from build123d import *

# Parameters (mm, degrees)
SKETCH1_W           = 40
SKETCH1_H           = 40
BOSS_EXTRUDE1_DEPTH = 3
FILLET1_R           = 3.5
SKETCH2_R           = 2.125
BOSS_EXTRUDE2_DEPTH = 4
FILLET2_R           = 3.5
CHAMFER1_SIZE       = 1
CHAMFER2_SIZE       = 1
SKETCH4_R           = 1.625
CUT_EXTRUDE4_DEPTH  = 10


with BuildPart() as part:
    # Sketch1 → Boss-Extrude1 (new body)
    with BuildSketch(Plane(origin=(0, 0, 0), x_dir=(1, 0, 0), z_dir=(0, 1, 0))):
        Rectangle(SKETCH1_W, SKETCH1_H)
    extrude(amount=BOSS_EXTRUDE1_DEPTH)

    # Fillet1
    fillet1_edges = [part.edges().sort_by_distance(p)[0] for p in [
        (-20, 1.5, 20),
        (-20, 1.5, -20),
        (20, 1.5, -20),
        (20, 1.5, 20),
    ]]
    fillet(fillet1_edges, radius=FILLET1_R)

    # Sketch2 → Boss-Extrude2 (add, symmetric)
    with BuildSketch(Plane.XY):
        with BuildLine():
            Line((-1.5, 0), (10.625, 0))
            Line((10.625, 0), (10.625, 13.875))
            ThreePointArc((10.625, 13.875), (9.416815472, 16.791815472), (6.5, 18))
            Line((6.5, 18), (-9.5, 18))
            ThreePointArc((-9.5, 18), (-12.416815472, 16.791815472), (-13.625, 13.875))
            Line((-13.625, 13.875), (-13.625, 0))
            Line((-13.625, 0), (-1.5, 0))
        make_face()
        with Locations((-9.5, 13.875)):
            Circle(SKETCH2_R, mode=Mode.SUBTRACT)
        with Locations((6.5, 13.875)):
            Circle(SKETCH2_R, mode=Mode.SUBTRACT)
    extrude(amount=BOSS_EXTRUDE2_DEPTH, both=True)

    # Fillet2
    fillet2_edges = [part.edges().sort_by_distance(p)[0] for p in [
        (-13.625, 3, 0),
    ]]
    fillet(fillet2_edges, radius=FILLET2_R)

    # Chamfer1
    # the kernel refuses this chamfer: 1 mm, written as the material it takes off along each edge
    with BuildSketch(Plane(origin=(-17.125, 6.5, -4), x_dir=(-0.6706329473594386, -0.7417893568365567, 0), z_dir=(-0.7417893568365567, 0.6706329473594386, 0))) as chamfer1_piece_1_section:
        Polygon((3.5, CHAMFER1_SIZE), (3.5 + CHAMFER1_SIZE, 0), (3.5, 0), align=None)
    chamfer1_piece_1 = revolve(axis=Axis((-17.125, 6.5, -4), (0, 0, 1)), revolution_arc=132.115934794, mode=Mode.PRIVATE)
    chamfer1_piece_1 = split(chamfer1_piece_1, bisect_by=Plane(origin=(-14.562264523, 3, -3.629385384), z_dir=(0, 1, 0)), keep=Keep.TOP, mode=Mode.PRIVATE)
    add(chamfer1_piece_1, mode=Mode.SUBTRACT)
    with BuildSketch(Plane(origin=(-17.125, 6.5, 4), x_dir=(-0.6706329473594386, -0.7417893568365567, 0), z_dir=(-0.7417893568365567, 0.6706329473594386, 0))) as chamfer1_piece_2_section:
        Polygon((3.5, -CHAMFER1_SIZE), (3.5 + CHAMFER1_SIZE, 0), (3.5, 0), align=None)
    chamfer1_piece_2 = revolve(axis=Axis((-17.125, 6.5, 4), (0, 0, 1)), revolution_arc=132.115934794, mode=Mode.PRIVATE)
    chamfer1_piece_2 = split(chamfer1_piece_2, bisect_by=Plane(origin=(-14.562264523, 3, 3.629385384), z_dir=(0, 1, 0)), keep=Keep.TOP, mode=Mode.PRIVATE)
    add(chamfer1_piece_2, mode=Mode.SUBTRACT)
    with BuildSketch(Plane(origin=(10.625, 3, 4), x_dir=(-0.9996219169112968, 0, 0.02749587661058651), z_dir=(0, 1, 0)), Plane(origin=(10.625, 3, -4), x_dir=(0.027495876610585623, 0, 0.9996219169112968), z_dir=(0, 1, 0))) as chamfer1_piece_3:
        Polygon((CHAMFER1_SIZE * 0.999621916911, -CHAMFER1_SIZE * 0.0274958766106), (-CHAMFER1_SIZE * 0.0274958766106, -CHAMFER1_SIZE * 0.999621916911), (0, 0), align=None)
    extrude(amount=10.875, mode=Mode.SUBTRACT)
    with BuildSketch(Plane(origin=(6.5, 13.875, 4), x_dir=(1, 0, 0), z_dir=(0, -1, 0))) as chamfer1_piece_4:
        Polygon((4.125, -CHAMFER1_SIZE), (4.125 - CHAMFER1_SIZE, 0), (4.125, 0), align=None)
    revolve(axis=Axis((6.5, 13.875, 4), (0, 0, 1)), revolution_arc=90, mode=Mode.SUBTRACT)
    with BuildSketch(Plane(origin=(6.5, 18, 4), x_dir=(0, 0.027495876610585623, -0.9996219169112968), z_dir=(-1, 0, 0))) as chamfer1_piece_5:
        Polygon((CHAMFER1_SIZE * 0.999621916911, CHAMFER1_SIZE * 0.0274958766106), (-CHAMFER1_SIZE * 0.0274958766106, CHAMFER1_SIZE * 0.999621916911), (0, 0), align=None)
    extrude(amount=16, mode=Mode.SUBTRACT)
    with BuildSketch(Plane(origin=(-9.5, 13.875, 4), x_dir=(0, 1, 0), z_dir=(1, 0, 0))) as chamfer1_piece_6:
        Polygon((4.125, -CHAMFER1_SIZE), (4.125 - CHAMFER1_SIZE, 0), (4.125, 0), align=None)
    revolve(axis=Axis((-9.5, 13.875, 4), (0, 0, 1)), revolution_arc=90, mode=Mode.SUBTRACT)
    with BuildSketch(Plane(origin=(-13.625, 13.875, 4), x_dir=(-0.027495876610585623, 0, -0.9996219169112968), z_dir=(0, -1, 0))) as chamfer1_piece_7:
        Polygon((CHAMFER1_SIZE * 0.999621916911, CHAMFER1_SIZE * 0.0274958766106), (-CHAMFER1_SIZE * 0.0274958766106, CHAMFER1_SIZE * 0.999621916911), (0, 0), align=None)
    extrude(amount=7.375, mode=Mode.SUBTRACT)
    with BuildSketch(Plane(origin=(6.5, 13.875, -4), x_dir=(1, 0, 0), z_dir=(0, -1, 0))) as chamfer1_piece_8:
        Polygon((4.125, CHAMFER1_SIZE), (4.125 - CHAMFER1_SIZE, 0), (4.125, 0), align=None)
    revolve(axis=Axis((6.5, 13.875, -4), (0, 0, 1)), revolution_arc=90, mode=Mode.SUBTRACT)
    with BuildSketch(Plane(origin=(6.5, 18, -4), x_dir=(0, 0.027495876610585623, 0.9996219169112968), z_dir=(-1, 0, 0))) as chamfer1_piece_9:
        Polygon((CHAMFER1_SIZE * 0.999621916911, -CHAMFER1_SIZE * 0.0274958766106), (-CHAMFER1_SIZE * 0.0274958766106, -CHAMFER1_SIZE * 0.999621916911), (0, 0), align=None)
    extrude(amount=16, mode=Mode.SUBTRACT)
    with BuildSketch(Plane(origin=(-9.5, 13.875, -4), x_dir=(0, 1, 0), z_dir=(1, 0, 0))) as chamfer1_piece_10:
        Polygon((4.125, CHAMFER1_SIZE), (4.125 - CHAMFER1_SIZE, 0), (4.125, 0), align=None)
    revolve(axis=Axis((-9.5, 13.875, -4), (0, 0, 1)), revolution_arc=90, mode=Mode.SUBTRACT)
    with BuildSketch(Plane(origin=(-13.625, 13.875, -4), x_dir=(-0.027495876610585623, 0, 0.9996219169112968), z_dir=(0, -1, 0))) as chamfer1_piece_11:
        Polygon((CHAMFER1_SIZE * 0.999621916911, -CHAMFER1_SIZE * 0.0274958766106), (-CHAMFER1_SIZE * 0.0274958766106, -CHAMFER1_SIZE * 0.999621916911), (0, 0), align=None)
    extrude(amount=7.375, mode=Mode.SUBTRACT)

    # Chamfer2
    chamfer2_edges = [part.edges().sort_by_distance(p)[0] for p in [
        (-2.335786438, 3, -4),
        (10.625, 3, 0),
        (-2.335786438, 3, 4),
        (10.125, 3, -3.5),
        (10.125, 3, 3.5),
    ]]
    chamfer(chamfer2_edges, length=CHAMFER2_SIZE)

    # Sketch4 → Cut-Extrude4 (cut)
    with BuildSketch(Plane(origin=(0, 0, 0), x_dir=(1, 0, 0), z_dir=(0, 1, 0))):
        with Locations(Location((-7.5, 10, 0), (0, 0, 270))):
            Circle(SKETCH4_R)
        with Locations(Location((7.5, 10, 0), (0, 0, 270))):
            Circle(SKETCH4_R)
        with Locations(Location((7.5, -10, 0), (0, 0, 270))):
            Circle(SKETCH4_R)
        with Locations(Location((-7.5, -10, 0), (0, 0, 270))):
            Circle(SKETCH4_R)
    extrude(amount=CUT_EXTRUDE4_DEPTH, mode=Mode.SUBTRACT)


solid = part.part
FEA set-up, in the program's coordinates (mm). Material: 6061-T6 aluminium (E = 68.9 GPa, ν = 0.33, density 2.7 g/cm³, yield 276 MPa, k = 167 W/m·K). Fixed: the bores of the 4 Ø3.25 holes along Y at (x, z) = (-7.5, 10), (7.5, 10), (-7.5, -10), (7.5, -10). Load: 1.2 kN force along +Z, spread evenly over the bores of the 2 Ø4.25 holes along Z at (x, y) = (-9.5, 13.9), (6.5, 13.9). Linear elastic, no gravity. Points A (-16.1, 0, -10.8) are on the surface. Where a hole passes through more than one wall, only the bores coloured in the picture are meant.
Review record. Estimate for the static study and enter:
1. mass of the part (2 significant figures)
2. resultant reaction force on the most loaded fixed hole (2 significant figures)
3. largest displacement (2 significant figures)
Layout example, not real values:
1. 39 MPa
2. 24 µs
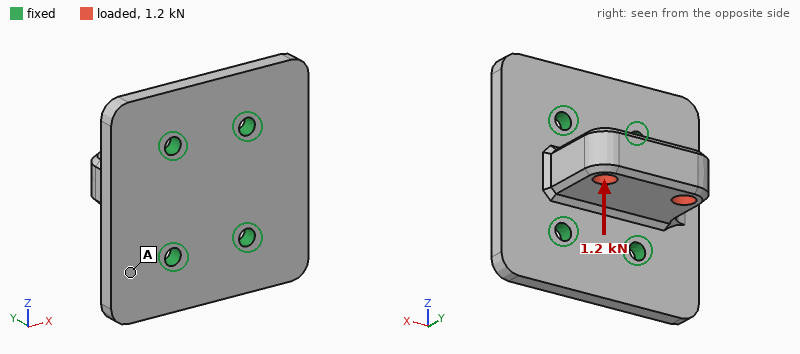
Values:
1. 20 g
2. 620 N
3. 36 µm
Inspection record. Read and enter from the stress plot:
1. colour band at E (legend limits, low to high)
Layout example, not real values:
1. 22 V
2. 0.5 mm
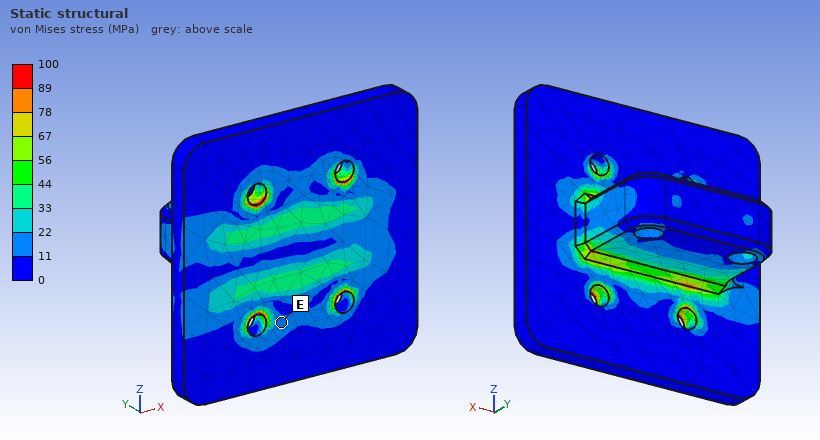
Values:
1. 11 to 22 MPa
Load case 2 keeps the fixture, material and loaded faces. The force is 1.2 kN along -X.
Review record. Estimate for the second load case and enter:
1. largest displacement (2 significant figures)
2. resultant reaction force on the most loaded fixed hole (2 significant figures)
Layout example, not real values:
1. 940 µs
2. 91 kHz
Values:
1. 25 µm
2. 530 N
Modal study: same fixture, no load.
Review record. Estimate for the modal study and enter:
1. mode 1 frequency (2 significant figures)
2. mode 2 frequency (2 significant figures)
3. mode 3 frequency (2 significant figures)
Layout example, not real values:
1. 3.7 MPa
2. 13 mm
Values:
1. 14 kHz
2. 17 kHz
3. 17 kHz
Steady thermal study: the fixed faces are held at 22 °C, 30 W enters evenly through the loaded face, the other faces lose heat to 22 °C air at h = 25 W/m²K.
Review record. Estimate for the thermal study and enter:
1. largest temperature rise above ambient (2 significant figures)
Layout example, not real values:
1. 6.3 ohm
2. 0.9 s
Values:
1. 22 K
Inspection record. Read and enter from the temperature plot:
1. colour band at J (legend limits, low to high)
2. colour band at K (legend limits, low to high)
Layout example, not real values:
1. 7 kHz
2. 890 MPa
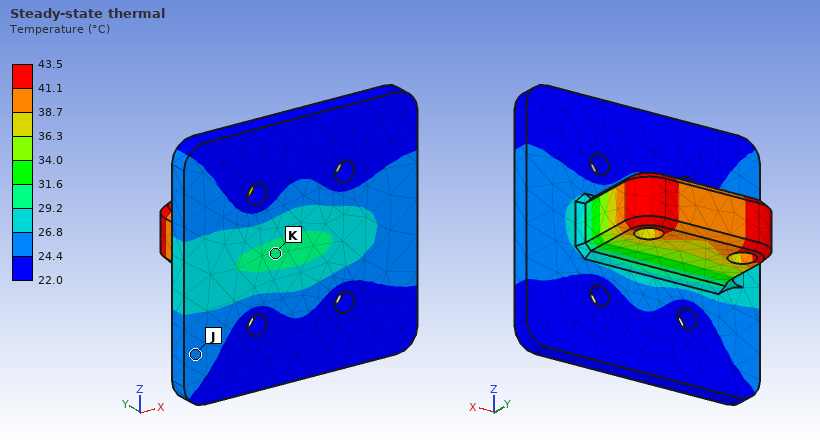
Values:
1. 24.4 to 26.8 °C
2. 29.2 to 31.6 °C
